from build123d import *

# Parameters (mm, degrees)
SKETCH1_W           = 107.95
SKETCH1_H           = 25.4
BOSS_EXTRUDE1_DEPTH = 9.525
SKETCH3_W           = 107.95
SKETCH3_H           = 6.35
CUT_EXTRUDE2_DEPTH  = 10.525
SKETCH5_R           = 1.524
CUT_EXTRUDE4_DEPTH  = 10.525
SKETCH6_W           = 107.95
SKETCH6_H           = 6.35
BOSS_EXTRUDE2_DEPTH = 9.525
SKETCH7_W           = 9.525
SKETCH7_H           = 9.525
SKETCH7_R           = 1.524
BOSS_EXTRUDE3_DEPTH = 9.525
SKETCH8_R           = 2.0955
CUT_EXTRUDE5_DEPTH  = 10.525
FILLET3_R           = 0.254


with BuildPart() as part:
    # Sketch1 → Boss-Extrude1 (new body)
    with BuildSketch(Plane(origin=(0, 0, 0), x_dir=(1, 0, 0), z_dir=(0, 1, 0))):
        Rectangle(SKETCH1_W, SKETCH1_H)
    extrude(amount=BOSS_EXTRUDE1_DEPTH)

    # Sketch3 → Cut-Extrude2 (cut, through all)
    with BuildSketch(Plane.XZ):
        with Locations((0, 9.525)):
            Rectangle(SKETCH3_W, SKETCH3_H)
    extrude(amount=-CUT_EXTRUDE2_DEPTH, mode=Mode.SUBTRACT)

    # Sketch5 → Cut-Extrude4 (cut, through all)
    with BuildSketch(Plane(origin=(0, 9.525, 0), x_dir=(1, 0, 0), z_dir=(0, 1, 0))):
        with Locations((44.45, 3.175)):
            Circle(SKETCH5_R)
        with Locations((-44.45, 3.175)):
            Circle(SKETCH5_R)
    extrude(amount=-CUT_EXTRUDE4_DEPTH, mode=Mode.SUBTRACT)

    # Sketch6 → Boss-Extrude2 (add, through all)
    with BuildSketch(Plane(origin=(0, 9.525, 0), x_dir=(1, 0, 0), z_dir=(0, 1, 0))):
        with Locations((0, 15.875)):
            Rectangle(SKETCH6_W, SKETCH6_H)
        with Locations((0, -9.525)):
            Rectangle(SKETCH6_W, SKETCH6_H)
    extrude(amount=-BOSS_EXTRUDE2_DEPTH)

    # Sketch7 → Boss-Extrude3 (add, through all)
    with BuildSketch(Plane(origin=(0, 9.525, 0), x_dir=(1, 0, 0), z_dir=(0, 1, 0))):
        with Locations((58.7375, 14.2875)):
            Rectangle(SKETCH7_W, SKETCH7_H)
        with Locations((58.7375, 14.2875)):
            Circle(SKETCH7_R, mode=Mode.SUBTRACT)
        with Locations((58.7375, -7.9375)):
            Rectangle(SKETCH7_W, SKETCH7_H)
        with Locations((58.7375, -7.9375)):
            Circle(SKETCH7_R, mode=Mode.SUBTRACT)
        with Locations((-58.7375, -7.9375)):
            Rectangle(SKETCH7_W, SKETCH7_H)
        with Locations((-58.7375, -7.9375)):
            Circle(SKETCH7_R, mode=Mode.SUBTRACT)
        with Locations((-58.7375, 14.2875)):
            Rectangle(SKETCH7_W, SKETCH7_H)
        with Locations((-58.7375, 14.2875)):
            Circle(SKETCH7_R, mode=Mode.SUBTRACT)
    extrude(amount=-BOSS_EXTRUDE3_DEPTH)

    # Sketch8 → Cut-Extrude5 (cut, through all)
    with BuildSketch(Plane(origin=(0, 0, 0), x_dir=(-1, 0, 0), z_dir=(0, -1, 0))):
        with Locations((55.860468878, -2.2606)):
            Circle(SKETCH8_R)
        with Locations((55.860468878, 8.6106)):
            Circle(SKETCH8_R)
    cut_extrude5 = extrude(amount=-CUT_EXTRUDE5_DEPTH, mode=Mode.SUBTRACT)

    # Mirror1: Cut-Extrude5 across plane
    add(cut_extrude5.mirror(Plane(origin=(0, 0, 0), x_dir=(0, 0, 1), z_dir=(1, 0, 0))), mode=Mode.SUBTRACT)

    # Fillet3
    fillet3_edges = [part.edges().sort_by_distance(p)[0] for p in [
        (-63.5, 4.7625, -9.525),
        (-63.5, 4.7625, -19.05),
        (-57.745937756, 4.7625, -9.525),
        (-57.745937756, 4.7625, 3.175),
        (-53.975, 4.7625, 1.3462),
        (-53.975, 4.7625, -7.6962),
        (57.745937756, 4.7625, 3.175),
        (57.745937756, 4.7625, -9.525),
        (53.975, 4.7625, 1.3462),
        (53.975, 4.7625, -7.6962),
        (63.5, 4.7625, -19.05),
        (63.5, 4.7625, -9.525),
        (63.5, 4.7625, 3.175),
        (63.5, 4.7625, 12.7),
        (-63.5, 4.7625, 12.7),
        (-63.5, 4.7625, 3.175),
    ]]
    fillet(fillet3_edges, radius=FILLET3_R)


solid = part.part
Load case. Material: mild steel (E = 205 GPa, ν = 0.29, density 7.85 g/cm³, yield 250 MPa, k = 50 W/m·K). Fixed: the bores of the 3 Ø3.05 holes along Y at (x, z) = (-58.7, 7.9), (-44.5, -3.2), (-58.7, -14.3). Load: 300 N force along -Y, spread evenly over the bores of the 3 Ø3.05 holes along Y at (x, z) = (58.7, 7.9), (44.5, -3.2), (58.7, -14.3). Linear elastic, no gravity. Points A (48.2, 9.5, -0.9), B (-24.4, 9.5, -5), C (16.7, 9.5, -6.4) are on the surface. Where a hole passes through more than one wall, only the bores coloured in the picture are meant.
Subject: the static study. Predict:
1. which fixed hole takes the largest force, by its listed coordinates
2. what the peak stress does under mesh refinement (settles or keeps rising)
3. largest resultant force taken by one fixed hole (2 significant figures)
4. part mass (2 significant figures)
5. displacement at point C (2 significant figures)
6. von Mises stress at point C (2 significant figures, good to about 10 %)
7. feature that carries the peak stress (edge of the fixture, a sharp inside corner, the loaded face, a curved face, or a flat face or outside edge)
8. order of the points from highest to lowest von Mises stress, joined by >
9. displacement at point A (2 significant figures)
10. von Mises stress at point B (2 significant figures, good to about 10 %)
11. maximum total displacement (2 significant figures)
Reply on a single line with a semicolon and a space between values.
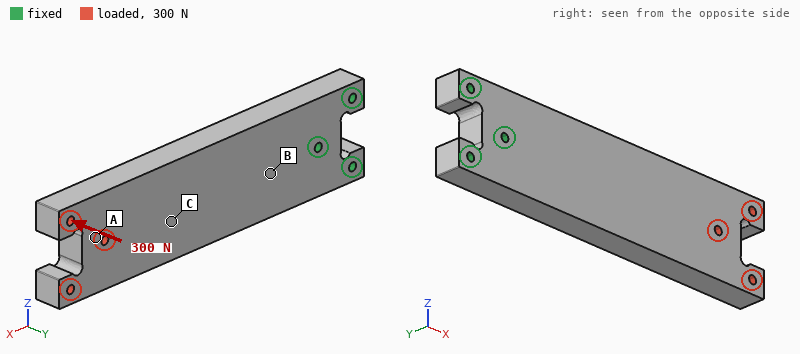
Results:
(-44.5, -3.2); keeps rising; 1.3 kN; 280 g; 0.11 mm; 23 MPa; edge of the fixture; B > C > A; 0.20 mm; 46 MPa; 0.25 mm
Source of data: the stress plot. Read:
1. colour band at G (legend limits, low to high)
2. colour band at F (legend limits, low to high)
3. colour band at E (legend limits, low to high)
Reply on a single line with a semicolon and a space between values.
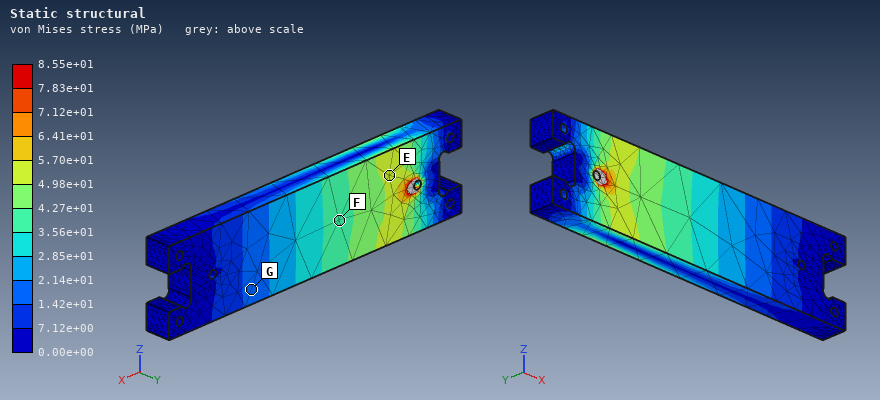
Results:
1.42e+01 to 2.14e+01 MPa; 3.56e+01 to 4.27e+01 MPa; 4.98e+01 to 5.70e+01 MPa
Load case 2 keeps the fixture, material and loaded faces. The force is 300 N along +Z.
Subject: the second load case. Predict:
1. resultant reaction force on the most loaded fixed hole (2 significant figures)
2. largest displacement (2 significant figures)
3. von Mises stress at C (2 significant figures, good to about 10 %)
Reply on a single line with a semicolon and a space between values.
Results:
1.0 kN; 32 µm; 2.9 MPa
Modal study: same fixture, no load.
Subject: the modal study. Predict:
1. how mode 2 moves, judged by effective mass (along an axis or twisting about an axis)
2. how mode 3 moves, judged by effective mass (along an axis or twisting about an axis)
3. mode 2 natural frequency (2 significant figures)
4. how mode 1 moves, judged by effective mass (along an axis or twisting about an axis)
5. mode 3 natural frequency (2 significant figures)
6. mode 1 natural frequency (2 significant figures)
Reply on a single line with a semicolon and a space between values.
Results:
along Z; twisting about X; 1900 Hz; along Y; 3800 Hz; 690 Hz
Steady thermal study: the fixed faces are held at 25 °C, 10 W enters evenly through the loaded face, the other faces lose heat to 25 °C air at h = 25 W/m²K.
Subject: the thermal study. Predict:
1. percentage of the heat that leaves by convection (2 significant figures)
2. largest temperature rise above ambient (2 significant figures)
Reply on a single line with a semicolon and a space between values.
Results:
51 %; 46 K
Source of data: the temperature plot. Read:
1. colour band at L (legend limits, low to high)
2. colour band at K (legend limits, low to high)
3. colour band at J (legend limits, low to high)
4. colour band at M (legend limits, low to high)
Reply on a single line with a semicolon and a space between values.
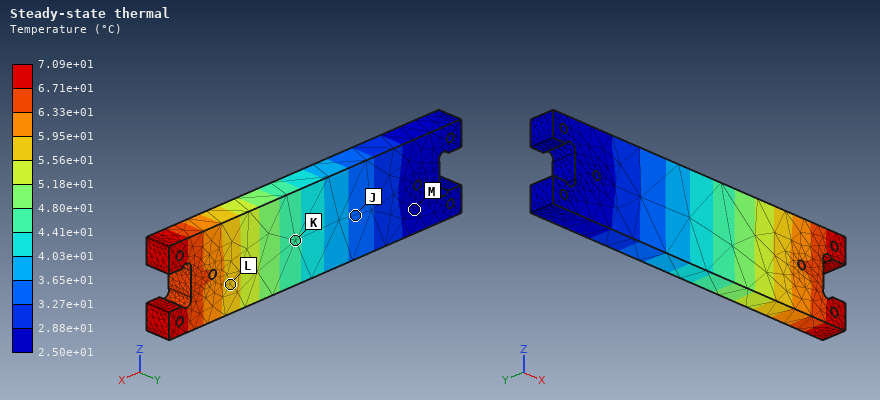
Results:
5.56e+01 to 5.95e+01 °C; 4.41e+01 to 4.80e+01 °C; 3.27e+01 to 3.65e+01 °C; 2.50e+01 to 2.88e+01 °C
